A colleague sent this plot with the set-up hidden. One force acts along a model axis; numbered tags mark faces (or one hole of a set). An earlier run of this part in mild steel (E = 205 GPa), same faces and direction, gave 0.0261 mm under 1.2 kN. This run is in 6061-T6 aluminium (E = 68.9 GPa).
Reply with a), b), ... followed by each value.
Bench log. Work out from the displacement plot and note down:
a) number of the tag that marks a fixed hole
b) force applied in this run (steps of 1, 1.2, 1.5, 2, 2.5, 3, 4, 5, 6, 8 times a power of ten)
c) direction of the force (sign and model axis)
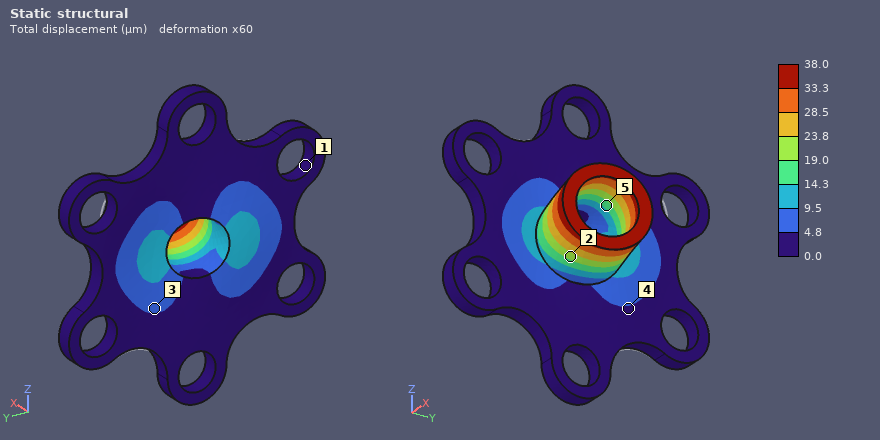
a) 1
b) 600 N
c) -Y
